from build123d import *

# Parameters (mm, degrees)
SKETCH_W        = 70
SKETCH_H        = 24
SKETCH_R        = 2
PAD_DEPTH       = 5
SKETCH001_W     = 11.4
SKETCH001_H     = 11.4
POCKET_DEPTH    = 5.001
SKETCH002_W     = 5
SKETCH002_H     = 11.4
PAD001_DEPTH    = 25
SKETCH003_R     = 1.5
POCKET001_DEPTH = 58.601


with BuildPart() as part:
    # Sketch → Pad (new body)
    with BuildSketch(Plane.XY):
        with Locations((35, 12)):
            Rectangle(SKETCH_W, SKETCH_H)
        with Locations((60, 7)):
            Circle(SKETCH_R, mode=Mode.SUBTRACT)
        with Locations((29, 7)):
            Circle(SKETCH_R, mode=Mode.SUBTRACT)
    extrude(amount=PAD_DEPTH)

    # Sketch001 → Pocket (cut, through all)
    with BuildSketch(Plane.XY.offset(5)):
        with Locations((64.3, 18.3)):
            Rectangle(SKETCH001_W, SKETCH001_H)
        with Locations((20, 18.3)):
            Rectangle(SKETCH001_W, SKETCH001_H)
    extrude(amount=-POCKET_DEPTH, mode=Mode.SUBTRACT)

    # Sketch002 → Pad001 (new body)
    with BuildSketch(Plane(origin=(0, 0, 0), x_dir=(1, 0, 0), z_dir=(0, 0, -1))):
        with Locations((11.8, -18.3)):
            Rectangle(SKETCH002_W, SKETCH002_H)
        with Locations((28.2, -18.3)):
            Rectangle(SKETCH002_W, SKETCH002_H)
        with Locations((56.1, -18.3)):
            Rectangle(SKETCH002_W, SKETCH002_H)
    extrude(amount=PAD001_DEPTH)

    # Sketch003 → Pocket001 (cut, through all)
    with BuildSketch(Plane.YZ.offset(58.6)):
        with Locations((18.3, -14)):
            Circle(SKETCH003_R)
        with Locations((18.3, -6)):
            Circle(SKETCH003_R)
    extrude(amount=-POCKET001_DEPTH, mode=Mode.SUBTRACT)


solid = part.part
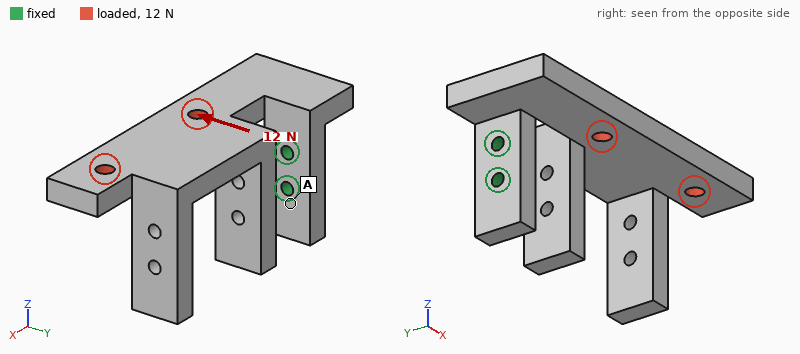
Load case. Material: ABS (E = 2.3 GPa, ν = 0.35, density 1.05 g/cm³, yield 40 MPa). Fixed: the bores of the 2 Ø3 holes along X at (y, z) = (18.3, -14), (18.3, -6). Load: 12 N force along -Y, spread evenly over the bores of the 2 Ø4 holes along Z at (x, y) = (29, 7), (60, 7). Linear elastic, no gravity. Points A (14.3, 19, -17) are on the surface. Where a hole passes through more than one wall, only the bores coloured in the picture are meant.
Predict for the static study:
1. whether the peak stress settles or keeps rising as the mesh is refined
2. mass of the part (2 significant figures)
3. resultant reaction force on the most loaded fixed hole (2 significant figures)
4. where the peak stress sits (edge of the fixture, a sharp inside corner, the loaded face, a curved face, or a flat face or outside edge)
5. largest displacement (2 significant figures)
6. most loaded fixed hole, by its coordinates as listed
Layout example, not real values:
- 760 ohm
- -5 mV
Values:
- keeps rising
- 12 g
- 19 N
- edge of the fixture
- 0.84 mm
- (18.3, -6)
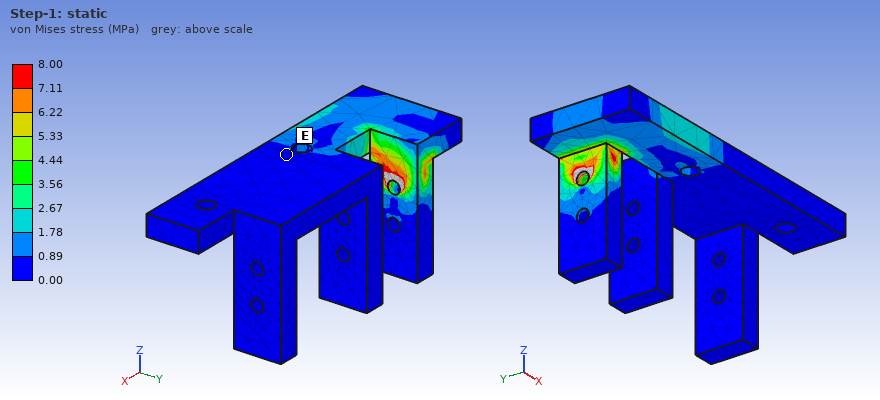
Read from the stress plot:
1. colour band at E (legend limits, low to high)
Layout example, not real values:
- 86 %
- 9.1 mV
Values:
- 0.00 to 0.89 MPa
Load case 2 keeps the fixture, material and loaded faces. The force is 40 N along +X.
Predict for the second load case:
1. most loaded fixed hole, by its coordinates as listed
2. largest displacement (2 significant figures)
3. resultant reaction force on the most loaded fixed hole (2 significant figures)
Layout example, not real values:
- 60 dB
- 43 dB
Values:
- (18.3, -6)
- 0.78 mm
- 48 N
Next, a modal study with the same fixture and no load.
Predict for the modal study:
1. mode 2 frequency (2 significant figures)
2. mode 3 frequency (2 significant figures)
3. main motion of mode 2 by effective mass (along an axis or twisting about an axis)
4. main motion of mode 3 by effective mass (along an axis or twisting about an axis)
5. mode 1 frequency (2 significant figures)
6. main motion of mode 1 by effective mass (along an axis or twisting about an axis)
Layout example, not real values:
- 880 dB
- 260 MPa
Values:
- 260 Hz
- 480 Hz
- along Y
- twisting about X
- 170 Hz
- along Z
